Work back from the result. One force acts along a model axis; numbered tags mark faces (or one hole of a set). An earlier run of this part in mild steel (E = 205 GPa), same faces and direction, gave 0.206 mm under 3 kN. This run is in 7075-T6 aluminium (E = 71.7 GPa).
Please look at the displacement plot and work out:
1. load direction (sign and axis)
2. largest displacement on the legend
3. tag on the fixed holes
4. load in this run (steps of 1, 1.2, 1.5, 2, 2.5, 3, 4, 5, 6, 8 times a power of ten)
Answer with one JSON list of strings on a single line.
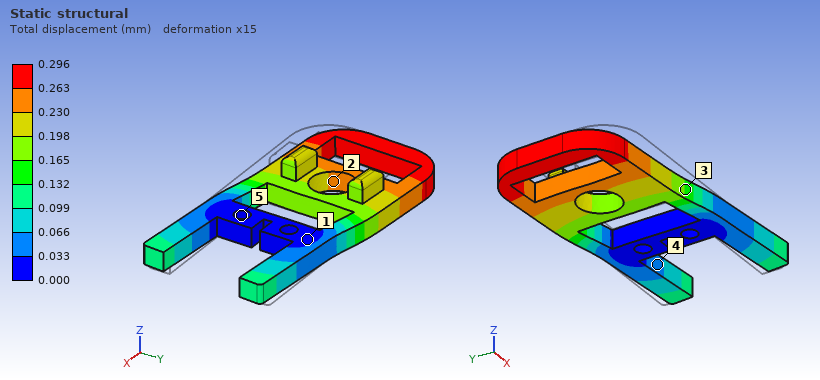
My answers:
["+Y", "0.296 mm", "5", "1.5 kN"]
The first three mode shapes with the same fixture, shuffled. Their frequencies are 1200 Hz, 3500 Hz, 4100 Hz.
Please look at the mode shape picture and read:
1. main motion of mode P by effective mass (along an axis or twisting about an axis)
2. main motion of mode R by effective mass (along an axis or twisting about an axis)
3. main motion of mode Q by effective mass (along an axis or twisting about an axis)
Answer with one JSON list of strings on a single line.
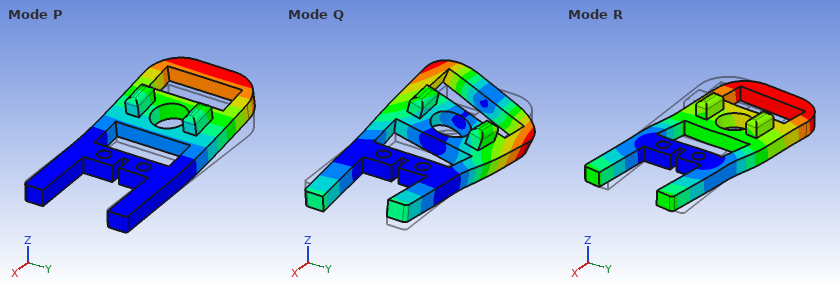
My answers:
["along Z", "along Y", "twisting about X"]
